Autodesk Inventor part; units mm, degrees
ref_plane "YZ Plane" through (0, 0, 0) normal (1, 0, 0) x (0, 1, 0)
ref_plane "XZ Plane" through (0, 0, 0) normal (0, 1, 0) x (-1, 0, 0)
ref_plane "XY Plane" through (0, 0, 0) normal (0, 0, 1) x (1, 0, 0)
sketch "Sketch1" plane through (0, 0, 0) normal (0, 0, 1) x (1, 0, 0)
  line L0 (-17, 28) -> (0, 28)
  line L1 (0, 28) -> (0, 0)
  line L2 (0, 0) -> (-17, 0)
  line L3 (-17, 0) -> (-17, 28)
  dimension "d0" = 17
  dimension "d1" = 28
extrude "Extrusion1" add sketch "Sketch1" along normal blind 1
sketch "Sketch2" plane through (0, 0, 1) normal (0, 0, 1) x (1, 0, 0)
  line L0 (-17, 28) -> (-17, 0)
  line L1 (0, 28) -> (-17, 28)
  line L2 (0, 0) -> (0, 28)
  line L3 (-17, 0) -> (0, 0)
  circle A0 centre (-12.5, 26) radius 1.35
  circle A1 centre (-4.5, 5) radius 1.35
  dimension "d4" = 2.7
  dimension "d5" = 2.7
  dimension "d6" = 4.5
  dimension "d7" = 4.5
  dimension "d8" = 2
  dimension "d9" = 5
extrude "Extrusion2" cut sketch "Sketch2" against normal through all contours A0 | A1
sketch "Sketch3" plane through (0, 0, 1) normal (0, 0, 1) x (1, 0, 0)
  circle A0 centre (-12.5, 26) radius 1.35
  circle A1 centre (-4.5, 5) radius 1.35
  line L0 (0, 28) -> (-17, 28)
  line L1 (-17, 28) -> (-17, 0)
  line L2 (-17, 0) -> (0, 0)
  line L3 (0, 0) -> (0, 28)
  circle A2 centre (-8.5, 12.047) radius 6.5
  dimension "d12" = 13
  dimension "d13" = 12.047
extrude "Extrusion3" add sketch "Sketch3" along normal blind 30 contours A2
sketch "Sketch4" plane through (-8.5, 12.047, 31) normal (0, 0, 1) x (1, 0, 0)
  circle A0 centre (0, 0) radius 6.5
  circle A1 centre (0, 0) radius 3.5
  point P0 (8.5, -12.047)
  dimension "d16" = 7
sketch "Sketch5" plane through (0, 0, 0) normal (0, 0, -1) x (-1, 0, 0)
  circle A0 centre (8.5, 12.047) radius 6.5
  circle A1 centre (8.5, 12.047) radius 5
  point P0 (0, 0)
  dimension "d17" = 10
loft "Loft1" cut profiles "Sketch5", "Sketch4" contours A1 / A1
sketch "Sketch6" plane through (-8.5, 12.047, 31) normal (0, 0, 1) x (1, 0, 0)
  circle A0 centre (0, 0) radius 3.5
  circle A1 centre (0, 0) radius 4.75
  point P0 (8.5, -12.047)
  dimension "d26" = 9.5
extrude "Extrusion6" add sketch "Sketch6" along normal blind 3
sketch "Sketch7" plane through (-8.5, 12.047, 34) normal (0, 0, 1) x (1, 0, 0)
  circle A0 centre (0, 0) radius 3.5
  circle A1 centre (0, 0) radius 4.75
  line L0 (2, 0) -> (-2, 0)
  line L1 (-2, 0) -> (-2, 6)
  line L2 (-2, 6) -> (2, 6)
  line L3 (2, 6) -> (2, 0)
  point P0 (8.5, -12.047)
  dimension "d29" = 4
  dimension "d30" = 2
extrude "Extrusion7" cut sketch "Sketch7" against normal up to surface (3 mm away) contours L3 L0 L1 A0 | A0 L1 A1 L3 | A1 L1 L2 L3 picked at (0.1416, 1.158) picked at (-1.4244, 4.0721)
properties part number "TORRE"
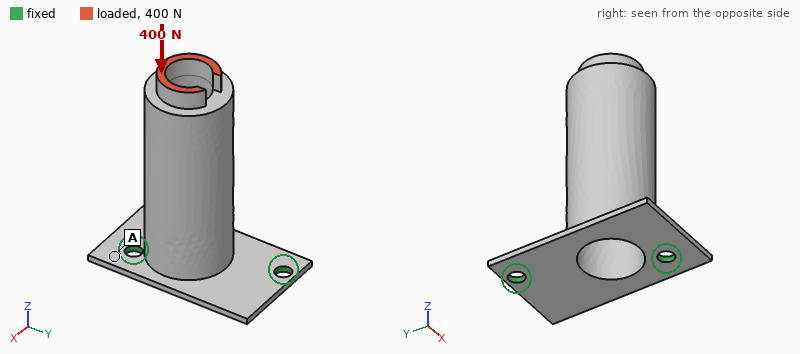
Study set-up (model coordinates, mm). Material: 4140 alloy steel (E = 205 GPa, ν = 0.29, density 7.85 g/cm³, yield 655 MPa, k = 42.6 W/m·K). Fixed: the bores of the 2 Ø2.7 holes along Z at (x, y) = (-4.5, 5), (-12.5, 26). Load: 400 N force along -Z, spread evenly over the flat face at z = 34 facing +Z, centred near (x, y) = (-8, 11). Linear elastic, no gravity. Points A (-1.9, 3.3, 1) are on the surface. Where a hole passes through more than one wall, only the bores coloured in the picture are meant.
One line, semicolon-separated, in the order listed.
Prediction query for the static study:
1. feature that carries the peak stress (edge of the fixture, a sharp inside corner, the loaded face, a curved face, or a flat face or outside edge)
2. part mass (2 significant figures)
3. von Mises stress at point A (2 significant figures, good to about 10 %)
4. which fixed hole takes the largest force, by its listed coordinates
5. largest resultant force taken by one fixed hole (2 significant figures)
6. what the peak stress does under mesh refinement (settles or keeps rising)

edge of the fixture; 22 g; 26 MPa; (-4.5, 5); 280 N; keeps rising
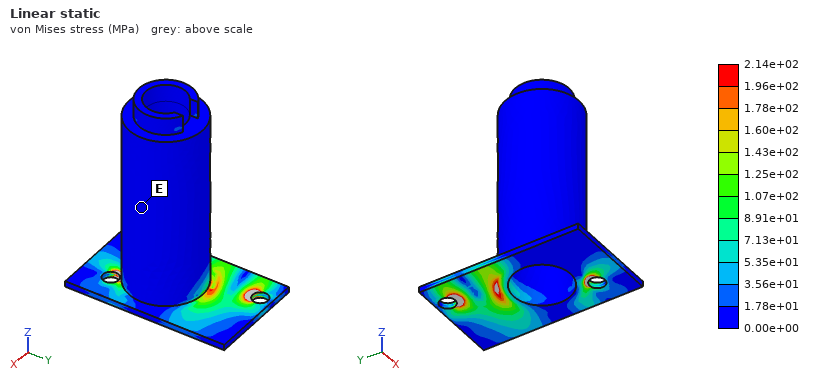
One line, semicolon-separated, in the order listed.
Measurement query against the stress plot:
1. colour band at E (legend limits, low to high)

0.00e+00 to 1.78e+01 MPa
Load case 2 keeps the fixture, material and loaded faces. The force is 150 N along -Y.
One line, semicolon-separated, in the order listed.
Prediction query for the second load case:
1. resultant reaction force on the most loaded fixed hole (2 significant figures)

260 N
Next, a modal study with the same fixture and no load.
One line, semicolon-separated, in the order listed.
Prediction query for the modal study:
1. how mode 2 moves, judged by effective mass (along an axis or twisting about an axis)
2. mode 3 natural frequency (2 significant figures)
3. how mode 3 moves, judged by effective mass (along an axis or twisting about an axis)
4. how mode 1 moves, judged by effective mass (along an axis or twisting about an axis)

along Y; 11 kHz; along Z; along X
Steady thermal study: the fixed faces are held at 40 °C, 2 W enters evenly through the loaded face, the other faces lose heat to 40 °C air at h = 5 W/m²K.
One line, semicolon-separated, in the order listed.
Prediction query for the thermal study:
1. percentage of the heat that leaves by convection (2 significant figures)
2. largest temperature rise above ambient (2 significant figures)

12 %; 33 K
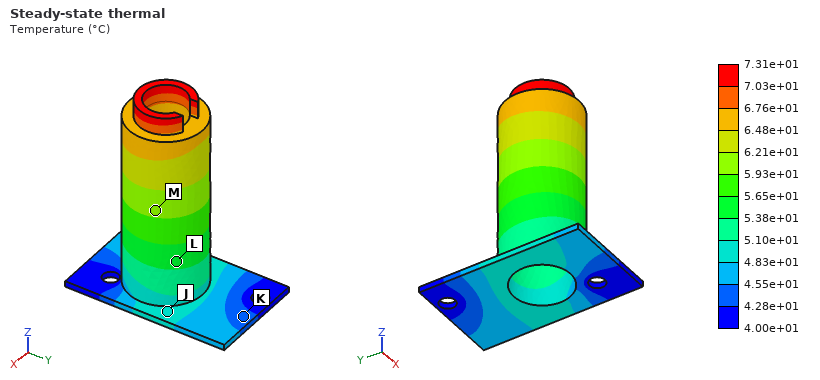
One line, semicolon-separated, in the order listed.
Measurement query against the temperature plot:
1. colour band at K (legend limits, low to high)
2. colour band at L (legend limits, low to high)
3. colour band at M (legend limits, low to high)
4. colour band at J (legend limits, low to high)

4.28e+01 to 4.55e+01 °C; 5.38e+01 to 5.65e+01 °C; 5.93e+01 to 6.21e+01 °C; 4.83e+01 to 5.10e+01 °C
